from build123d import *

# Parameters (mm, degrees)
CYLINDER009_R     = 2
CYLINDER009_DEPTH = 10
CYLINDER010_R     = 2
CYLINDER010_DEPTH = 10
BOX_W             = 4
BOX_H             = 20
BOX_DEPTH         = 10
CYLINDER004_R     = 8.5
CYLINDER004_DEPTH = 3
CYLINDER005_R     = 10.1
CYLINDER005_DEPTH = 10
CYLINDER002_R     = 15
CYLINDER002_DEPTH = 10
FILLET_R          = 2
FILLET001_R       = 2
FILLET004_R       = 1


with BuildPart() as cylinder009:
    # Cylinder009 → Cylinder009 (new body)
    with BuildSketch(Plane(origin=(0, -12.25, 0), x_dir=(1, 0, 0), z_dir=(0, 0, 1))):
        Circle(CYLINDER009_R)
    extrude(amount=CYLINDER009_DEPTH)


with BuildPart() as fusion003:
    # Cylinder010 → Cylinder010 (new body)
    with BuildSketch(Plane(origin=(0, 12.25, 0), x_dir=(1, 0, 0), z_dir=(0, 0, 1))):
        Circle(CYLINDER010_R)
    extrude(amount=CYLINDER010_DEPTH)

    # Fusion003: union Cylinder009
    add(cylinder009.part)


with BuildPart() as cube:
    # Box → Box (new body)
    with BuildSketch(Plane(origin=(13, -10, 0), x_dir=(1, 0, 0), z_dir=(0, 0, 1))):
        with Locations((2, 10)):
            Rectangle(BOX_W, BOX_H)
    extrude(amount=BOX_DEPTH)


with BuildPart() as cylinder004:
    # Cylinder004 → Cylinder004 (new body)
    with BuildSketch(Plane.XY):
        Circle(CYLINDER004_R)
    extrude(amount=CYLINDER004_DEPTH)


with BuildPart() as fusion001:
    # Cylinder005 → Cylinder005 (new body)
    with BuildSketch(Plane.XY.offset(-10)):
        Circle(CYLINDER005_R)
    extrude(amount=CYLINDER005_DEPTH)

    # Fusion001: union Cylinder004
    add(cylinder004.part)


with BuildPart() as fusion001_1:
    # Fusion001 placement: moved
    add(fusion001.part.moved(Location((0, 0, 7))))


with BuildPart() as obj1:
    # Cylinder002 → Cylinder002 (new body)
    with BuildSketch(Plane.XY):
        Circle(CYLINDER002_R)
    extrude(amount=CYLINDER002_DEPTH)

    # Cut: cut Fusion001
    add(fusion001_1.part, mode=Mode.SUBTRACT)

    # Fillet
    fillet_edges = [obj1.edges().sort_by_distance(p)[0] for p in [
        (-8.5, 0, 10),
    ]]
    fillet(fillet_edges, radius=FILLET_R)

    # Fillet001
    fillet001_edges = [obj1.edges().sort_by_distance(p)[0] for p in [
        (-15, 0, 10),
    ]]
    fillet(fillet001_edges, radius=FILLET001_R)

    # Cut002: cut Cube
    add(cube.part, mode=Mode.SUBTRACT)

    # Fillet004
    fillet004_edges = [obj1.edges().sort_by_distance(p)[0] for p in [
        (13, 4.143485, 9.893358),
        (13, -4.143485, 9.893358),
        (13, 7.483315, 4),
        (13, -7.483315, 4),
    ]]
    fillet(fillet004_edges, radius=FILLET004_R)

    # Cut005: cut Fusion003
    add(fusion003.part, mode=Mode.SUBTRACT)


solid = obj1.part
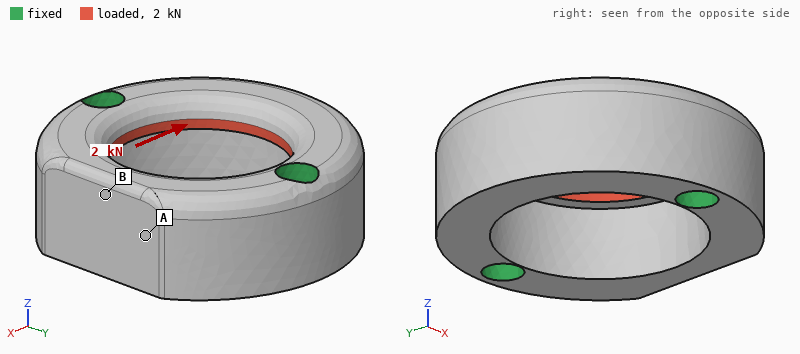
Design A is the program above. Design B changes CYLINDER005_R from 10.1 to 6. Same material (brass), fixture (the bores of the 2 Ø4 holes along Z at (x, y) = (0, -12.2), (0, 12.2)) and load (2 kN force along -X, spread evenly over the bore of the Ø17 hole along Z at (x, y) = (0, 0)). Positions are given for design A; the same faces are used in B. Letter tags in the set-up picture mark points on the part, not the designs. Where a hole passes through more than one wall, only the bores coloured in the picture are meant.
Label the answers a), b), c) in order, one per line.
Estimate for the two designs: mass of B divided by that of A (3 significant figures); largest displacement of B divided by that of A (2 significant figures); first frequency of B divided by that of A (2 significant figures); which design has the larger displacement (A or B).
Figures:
a) 1.41
b) 0.70
c) 1.1
d) A
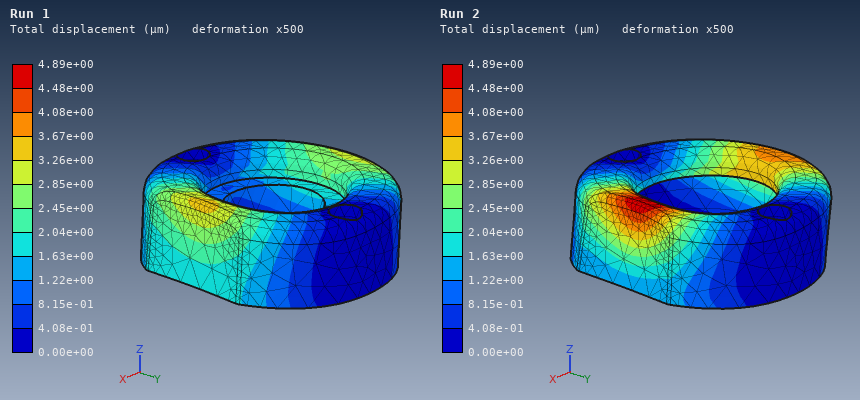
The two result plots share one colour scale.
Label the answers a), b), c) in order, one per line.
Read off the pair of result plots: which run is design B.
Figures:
a) Run 1
